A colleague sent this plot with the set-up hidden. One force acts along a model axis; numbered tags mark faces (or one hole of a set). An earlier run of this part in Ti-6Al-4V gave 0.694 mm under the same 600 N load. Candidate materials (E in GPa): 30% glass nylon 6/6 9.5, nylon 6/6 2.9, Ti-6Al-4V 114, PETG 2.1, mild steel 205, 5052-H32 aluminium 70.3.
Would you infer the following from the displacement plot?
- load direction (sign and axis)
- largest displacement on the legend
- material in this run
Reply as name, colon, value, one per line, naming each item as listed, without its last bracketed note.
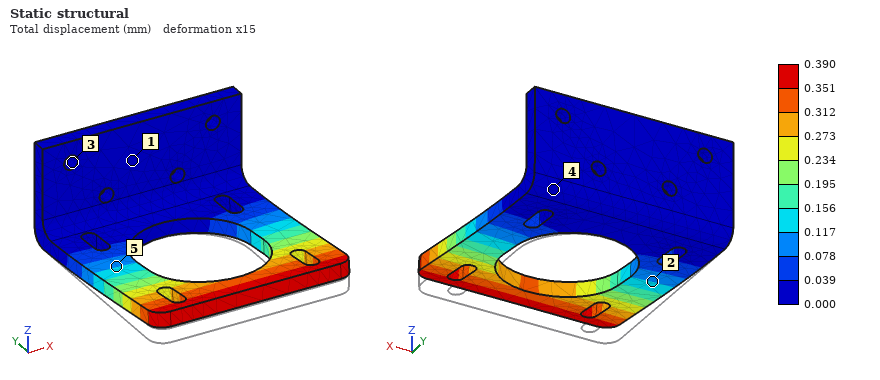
load direction: +Z
largest displacement on the legend: 0.390 mm
material in this run: mild steel
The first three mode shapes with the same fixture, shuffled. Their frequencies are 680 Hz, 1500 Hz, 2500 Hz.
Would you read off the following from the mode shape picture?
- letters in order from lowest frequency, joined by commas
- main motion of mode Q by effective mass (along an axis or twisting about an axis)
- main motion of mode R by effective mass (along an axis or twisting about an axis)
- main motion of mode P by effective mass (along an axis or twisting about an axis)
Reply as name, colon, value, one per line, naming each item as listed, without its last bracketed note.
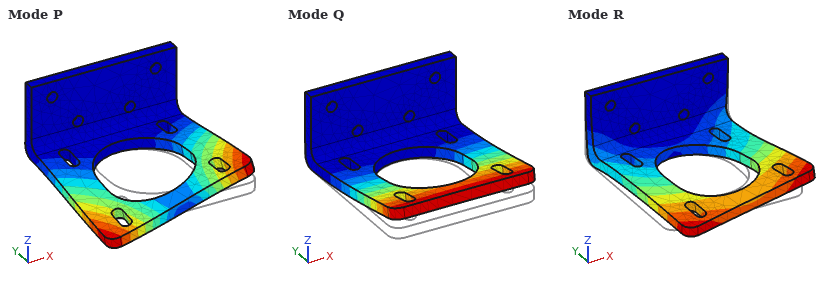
letters in order from lowest frequency, joined by commas: Q, P, R
main motion of mode Q by effective mass: along Z
main motion of mode R by effective mass: along X
main motion of mode P by effective mass: twisting about Y
